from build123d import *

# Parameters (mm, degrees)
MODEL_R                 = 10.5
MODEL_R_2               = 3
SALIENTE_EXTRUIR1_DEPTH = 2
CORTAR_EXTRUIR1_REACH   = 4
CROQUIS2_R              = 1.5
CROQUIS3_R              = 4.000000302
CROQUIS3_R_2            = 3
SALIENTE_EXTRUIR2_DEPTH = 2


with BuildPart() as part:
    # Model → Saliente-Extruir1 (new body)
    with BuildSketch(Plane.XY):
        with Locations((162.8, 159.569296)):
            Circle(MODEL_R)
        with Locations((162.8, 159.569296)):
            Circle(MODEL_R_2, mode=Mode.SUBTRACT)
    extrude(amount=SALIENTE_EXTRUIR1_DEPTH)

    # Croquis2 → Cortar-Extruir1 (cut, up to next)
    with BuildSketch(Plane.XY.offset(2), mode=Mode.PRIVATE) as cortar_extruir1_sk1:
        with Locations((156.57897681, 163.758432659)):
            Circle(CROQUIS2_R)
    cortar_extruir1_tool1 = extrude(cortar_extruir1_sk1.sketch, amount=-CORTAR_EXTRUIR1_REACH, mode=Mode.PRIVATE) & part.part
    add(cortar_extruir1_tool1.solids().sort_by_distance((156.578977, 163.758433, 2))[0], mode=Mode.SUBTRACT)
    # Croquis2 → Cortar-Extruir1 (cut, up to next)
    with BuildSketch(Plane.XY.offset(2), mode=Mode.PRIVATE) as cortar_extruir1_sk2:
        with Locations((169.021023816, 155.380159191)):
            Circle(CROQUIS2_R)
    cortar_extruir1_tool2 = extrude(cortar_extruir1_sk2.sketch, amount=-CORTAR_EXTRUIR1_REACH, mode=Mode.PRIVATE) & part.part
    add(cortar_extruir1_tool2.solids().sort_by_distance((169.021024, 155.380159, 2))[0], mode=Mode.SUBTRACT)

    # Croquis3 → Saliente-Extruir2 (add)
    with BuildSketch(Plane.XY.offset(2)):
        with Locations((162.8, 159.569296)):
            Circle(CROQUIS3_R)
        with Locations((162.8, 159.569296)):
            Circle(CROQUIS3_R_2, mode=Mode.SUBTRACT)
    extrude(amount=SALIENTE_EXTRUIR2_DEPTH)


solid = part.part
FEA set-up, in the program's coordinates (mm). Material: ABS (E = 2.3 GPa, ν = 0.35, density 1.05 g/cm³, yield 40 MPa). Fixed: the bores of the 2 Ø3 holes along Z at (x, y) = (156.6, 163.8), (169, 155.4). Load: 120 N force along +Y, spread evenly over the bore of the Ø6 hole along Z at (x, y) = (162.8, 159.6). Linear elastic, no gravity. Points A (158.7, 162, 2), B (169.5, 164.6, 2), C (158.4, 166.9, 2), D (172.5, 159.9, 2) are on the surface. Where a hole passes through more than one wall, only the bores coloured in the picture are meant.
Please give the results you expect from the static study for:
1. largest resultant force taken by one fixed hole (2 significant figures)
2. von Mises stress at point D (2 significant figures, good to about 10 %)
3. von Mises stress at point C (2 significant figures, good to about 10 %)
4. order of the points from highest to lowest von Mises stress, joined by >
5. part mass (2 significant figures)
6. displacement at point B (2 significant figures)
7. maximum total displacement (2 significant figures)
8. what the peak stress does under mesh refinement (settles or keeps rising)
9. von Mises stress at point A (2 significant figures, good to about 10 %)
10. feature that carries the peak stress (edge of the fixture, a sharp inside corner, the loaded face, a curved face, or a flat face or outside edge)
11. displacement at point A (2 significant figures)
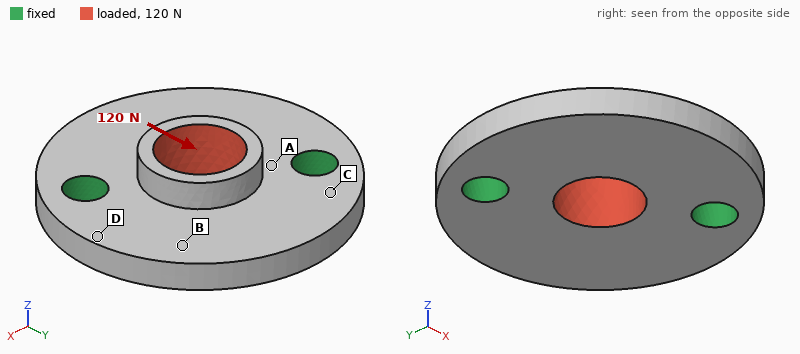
60 N
2.1 MPa
3.8 MPa
A > C > D > B
0.68 g
39 µm
55 µm
keeps rising
9.2 MPa
edge of the fixture
8.9 µm
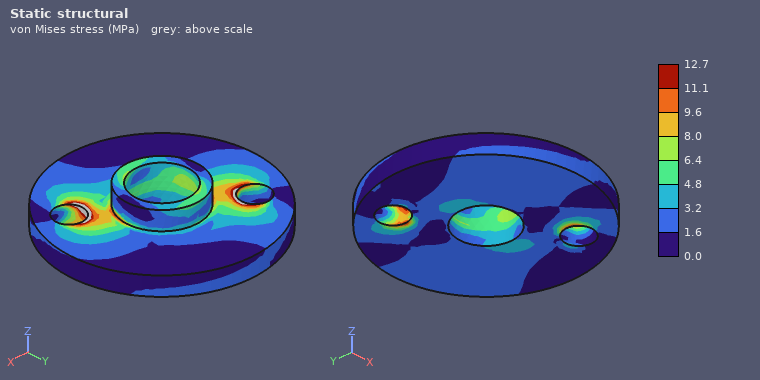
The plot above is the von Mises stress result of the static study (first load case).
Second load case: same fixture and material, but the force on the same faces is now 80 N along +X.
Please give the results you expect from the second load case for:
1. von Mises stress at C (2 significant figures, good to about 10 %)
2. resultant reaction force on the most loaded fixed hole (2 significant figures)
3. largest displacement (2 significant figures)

1.7 MPa
40 N
25 µm
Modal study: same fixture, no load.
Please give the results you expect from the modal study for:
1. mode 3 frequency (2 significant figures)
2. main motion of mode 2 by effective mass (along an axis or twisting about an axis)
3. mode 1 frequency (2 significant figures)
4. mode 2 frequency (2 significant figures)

12 kHz
along Z
5100 Hz
5900 Hz
